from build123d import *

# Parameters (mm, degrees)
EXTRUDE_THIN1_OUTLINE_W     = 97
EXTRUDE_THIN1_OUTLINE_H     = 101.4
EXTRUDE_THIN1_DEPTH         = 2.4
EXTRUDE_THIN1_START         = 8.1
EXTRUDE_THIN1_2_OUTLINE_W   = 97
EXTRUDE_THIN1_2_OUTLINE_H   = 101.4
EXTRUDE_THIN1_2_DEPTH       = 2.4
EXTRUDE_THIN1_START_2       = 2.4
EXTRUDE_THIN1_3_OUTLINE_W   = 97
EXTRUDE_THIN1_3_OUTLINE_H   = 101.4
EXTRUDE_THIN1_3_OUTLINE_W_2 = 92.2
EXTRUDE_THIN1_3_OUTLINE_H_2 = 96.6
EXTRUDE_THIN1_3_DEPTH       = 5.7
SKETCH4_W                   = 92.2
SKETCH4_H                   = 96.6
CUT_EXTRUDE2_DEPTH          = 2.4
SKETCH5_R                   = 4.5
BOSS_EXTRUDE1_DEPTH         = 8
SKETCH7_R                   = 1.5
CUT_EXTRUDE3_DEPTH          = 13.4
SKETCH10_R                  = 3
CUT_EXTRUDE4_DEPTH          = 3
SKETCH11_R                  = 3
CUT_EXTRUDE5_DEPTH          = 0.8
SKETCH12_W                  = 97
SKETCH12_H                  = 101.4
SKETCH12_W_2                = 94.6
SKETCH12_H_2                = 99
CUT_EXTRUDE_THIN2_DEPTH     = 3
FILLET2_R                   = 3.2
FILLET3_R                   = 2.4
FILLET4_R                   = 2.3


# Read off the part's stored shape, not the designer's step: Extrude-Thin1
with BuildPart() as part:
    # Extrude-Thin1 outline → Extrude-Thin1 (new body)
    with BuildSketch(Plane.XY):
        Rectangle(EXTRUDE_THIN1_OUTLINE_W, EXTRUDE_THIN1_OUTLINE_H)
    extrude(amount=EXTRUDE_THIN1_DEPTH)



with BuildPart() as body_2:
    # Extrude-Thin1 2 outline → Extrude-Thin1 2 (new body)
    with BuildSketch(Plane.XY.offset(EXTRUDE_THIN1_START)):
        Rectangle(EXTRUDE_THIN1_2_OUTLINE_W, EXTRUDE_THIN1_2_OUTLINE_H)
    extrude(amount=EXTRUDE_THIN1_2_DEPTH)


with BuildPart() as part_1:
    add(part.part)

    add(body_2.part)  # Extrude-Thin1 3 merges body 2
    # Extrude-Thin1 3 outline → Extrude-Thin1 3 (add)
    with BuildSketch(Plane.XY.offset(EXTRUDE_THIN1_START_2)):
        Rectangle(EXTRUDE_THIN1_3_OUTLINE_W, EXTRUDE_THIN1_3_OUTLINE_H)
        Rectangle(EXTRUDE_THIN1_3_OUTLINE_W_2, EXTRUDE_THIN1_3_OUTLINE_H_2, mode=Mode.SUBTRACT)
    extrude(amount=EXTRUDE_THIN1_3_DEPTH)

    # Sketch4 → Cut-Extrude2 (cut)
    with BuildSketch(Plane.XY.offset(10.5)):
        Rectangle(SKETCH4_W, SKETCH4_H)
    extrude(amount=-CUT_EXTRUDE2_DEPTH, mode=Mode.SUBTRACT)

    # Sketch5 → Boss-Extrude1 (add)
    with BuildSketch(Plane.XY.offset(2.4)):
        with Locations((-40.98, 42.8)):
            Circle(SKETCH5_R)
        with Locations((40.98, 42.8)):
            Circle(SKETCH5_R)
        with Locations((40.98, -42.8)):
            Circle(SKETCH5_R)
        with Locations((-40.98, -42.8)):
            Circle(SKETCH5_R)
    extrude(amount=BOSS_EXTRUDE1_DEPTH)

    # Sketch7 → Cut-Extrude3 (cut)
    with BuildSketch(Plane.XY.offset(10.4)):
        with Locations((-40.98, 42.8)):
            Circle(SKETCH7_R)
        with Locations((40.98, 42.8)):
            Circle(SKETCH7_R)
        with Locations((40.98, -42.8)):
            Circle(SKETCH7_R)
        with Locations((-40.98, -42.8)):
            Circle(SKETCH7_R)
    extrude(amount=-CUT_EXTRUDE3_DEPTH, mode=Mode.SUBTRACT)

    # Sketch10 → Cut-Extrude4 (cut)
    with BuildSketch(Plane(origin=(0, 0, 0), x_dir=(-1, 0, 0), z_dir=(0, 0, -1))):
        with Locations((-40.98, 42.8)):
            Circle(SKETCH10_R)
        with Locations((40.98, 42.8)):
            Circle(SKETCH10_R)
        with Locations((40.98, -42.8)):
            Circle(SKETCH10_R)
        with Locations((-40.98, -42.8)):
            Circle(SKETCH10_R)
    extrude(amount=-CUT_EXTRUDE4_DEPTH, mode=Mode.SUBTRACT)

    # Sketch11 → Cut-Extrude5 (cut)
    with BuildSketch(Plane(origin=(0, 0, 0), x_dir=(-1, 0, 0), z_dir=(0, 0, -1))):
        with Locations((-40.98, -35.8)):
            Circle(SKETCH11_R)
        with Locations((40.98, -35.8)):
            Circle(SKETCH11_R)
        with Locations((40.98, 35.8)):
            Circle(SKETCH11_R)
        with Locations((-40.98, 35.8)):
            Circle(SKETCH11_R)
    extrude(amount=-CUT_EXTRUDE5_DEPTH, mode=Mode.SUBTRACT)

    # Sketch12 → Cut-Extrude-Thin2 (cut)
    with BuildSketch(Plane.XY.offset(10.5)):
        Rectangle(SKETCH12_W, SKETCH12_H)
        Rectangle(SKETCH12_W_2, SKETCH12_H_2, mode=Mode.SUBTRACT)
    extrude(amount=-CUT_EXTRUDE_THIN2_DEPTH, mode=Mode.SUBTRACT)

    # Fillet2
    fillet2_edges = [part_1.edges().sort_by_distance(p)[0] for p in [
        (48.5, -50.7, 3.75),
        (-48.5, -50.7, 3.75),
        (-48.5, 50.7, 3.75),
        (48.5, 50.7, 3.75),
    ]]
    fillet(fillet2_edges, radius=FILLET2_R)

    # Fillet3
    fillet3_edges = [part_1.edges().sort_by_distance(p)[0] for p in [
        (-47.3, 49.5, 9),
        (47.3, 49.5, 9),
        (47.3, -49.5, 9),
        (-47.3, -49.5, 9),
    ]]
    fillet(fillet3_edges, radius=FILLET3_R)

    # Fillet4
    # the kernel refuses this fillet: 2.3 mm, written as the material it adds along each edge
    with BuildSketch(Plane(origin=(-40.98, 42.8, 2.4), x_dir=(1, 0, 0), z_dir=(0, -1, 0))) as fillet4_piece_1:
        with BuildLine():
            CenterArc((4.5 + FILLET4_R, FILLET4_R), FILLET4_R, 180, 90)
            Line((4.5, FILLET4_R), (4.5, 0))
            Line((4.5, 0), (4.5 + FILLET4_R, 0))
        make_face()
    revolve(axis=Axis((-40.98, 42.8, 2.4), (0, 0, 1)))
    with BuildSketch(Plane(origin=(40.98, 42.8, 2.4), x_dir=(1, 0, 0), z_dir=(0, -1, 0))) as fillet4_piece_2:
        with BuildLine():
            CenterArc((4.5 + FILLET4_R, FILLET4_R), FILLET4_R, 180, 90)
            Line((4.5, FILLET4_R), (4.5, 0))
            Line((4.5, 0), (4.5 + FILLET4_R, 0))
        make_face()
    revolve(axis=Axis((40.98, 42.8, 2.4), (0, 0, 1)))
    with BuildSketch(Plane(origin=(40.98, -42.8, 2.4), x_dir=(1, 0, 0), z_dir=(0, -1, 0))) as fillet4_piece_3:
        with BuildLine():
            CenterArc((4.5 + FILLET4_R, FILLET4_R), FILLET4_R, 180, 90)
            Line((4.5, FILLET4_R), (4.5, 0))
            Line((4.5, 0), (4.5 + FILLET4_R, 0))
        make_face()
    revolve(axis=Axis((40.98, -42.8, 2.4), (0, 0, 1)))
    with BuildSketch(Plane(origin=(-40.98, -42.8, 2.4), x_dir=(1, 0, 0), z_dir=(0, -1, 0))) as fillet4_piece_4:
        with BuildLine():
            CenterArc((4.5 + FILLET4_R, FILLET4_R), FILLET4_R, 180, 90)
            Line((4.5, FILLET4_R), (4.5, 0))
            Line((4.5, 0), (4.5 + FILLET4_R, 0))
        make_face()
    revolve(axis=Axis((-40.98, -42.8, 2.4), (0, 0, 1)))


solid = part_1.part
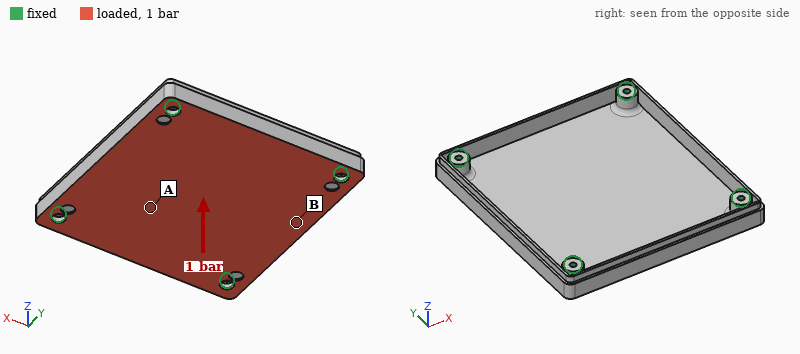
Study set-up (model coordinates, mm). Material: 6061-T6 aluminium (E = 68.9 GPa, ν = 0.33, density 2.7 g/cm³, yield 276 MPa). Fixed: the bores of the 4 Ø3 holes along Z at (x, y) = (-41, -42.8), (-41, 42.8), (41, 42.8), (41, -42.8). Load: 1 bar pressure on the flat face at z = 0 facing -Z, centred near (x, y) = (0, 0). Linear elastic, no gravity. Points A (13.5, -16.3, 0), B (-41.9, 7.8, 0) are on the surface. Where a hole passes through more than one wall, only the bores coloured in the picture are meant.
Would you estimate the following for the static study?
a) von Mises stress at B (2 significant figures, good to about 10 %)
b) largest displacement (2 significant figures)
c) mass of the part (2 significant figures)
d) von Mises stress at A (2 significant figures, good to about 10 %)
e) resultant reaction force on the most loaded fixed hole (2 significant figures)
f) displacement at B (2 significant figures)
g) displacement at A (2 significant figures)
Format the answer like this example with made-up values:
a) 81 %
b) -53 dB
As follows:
a) 16 MPa
b) 0.26 mm
c) 84 g
d) 29 MPa
e) 400 N
f) 0.068 mm
g) 0.21 mm
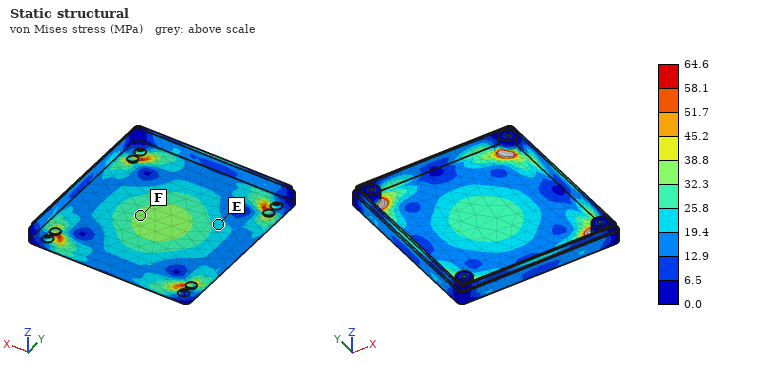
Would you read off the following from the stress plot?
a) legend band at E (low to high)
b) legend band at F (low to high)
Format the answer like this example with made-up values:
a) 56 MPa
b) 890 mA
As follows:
a) 19.4 to 25.8 MPa
b) 32.3 to 38.8 MPa
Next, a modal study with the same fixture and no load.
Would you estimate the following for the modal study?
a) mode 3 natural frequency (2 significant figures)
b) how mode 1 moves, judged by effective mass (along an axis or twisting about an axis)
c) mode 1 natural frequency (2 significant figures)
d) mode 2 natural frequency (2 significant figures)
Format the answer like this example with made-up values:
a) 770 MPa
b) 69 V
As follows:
a) 3100 Hz
b) along Z
c) 1500 Hz
d) 3100 Hz
